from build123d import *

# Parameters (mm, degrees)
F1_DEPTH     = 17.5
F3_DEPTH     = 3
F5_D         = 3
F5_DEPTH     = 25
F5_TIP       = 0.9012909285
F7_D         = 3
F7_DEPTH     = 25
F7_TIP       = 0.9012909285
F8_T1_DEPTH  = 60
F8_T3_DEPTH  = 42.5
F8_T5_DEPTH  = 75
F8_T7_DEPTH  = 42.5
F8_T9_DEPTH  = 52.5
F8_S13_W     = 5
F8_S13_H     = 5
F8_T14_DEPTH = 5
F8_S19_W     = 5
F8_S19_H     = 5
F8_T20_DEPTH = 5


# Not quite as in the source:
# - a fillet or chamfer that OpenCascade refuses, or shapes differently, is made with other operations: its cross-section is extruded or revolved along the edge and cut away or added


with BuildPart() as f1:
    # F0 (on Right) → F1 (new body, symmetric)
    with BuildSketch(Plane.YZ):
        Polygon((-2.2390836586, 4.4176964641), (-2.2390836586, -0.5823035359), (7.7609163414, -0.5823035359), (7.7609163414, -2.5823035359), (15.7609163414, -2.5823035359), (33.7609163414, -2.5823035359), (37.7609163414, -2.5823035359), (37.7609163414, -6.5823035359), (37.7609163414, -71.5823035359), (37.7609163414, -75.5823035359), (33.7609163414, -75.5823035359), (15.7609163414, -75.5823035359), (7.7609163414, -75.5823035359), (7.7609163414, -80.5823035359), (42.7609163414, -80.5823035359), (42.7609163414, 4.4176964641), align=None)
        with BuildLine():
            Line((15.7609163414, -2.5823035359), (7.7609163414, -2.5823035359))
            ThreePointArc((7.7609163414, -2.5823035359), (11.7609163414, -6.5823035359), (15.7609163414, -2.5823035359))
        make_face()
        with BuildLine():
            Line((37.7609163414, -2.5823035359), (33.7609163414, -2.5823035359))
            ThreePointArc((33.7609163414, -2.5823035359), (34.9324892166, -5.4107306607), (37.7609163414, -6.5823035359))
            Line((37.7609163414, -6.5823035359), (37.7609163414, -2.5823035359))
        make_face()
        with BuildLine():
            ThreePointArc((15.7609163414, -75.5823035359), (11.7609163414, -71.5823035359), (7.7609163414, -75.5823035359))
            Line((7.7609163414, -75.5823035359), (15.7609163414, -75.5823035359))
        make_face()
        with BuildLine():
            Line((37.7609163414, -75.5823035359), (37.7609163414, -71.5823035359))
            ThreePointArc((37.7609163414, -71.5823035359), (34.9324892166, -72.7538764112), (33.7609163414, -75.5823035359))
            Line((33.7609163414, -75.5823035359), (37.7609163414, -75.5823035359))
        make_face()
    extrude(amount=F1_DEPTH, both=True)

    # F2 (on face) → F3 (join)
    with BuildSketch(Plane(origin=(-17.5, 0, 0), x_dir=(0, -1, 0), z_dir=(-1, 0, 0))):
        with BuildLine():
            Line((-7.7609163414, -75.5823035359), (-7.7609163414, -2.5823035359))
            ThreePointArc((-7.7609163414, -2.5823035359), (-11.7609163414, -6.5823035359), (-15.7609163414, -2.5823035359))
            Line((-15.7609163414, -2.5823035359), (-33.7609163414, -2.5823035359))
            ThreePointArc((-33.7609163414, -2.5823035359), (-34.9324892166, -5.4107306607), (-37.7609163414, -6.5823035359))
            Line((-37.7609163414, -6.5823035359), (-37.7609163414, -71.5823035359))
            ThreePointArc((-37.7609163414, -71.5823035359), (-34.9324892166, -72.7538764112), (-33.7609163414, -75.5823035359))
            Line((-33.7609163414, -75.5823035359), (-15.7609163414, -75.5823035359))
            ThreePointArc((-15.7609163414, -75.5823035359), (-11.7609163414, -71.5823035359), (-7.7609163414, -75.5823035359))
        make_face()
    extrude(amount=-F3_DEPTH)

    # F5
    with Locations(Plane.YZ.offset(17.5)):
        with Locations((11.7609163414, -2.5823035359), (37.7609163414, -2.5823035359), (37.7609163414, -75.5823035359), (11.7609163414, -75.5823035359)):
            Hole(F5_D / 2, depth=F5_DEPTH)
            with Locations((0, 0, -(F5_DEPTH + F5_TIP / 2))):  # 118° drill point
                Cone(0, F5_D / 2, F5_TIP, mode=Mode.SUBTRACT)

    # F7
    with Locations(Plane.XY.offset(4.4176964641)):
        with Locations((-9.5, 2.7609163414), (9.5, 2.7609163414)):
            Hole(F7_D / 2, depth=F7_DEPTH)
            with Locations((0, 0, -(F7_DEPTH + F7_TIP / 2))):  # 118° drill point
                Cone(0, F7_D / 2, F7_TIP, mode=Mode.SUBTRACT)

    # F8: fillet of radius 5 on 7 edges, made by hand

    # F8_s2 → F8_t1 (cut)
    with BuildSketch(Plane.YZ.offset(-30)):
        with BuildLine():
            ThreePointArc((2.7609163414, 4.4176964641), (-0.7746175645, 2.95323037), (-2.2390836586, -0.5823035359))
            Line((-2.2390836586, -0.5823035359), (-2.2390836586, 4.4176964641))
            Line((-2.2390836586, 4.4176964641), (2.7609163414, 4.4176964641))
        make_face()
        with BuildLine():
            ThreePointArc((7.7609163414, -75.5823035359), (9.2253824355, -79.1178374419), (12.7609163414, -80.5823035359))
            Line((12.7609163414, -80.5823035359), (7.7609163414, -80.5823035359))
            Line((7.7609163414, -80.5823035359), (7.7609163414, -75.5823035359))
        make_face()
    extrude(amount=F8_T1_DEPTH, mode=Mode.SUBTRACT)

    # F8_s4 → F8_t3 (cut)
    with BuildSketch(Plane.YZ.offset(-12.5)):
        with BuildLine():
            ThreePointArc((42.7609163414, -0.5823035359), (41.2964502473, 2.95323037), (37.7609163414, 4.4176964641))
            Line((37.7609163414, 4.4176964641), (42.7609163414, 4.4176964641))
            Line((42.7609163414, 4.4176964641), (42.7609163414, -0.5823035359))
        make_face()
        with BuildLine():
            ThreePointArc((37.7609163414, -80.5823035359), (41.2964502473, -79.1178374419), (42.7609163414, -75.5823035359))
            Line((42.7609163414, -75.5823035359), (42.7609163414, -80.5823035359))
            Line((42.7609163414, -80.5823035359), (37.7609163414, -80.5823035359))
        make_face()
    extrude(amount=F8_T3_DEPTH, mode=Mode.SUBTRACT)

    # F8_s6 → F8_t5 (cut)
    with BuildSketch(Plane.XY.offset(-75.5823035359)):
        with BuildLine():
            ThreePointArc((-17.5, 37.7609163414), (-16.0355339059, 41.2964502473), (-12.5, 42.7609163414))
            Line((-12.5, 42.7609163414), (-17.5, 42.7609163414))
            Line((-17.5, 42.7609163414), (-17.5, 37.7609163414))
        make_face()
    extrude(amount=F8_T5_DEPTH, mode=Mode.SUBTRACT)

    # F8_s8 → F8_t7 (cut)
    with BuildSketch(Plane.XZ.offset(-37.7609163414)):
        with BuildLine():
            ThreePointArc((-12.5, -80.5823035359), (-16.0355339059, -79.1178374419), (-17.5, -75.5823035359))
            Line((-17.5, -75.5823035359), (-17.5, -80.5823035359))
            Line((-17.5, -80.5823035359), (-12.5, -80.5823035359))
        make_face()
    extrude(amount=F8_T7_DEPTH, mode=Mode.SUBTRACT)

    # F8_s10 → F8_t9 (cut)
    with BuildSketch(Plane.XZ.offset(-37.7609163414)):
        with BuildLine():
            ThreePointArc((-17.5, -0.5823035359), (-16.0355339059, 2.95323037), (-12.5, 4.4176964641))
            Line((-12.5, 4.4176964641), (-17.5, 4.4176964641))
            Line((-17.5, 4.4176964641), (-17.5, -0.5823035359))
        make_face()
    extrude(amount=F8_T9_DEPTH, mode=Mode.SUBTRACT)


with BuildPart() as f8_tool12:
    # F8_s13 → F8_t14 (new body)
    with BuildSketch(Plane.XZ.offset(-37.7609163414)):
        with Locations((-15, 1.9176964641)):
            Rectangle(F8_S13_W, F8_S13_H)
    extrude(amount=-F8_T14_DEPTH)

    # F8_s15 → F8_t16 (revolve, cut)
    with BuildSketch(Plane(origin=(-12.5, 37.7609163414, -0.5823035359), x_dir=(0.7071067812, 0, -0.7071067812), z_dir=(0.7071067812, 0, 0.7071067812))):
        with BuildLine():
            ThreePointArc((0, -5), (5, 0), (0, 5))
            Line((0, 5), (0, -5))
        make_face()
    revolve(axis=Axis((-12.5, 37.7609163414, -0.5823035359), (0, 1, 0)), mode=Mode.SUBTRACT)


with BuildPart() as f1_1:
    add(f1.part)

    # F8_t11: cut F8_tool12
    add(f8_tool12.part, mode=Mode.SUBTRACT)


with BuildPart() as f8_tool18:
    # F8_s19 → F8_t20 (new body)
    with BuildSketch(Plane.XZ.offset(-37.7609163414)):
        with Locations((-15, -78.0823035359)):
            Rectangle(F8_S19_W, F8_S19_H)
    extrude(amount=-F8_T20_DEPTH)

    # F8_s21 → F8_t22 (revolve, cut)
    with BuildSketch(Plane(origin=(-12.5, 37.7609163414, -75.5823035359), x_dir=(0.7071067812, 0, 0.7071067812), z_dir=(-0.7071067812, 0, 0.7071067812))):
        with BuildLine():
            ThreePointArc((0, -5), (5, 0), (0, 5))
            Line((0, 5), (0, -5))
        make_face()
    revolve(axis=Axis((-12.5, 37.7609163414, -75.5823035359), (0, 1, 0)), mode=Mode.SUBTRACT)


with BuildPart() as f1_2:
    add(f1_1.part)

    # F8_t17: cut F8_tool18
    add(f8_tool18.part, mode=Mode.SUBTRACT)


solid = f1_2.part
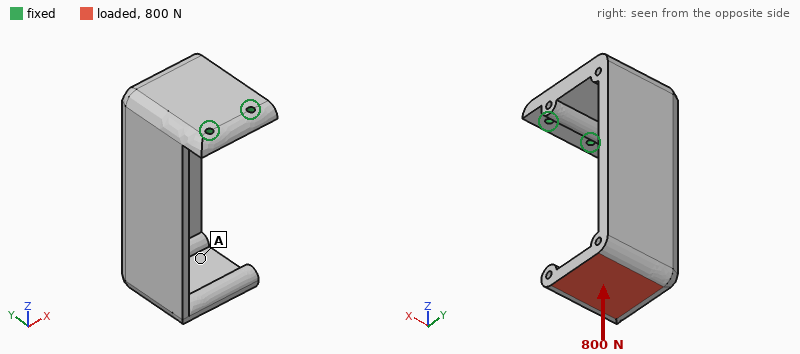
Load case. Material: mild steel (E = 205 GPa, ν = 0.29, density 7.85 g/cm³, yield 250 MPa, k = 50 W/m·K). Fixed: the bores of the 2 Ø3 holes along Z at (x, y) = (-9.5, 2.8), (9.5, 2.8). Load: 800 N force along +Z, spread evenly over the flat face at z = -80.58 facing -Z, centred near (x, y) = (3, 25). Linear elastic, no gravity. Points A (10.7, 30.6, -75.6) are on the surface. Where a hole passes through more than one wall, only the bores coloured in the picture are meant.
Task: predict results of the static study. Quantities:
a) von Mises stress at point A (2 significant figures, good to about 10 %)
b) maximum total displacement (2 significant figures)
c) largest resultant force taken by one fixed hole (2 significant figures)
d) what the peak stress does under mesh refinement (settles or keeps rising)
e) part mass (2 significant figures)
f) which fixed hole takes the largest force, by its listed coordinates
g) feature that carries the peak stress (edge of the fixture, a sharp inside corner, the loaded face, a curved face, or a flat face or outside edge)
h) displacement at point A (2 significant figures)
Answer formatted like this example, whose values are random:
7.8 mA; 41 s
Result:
21 MPa; 0.18 mm; 490 N; keeps rising; 280 g; (9.5, 2.8); edge of the fixture; 0.17 mm
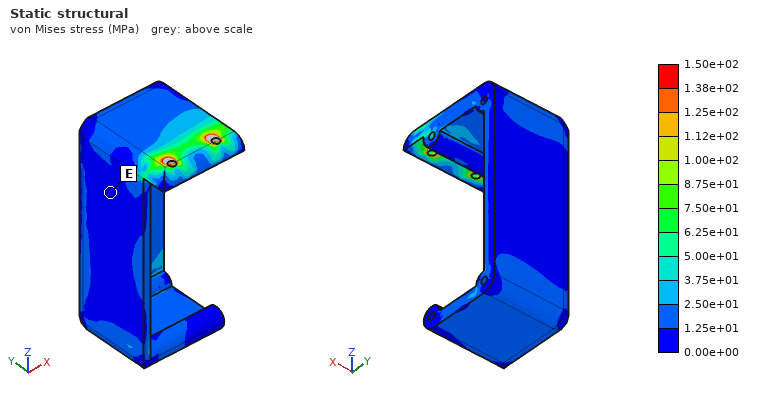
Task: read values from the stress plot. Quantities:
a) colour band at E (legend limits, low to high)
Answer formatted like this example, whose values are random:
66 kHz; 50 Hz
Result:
0.00e+00 to 1.25e+01 MPa
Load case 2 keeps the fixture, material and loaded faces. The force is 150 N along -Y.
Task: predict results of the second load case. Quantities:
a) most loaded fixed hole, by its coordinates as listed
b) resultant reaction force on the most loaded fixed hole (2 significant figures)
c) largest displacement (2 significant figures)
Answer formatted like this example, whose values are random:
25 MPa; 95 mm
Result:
(9.5, 2.8); 150 N; 0.22 mm
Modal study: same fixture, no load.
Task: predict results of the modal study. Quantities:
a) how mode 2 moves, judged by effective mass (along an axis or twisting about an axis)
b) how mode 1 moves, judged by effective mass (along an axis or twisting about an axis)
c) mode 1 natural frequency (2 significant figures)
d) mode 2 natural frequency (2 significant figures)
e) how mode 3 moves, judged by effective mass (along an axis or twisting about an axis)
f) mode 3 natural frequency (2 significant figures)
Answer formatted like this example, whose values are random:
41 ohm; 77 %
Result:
along X; along Y; 420 Hz; 630 Hz; along Z; 1600 Hz
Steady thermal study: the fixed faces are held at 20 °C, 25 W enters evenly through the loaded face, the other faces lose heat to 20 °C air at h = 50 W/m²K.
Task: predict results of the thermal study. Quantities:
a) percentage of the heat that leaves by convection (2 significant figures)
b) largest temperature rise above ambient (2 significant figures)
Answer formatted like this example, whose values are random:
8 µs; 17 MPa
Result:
88 %; 76 K
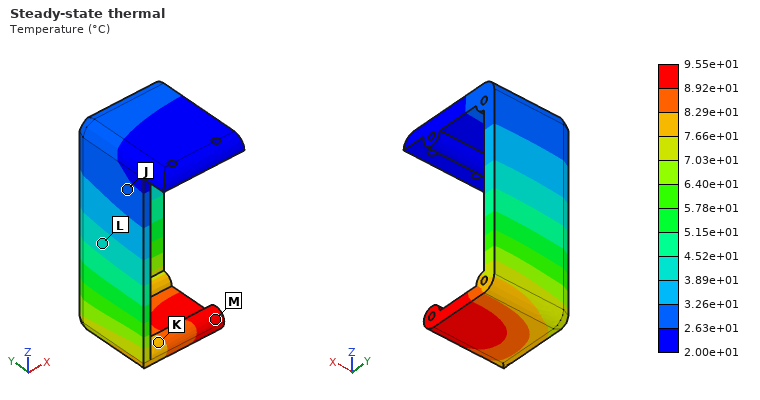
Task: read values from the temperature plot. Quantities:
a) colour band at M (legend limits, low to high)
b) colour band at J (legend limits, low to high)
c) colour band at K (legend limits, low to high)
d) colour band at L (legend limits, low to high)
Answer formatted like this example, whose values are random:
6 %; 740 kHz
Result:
8.92e+01 to 9.55e+01 °C; 2.63e+01 to 3.26e+01 °C; 7.66e+01 to 8.29e+01 °C; 3.89e+01 to 4.52e+01 °C
